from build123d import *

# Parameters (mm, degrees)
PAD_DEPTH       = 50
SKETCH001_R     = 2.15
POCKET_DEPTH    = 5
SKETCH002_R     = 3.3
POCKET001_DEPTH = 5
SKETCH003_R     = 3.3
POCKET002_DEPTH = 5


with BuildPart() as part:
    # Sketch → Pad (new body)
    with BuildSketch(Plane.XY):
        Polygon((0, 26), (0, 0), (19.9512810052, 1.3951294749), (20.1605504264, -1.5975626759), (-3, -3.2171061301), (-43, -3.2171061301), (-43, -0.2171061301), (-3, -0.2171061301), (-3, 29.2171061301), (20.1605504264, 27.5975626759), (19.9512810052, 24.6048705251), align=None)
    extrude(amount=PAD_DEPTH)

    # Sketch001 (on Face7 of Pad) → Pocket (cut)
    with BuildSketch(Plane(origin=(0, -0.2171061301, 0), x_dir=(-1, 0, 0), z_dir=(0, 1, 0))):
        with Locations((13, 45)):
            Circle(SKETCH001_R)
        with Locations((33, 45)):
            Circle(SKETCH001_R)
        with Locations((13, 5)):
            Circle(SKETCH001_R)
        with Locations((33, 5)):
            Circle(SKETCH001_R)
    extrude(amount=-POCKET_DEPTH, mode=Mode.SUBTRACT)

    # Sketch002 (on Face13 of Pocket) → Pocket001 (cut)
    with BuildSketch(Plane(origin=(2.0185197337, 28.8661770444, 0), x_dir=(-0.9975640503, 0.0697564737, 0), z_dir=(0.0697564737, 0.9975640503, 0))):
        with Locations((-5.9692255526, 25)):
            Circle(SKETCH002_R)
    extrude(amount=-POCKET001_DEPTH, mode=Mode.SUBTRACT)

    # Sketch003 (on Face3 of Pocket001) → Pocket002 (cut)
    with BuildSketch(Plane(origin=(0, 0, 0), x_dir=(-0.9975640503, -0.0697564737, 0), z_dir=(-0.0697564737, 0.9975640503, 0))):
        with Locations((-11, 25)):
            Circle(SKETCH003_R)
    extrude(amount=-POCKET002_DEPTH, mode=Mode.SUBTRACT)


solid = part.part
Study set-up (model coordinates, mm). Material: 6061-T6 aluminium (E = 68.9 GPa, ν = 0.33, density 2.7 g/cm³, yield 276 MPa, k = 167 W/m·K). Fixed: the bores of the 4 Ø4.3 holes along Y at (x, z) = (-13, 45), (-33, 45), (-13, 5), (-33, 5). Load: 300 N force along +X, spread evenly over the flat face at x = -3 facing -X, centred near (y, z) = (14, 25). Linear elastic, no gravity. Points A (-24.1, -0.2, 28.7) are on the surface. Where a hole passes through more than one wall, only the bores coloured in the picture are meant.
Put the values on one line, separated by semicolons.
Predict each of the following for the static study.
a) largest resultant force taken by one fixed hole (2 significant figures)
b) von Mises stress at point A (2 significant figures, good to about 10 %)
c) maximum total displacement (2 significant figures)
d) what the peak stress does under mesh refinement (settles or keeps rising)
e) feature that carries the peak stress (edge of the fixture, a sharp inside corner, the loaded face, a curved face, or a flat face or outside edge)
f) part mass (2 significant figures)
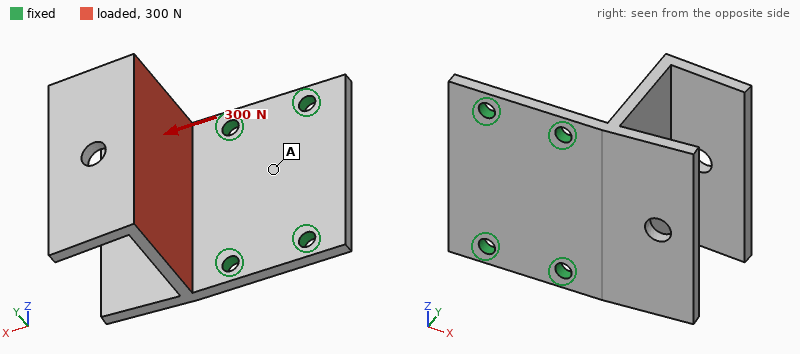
120 N; 9.0 MPa; 0.44 mm; keeps rising; edge of the fixture; 45 g
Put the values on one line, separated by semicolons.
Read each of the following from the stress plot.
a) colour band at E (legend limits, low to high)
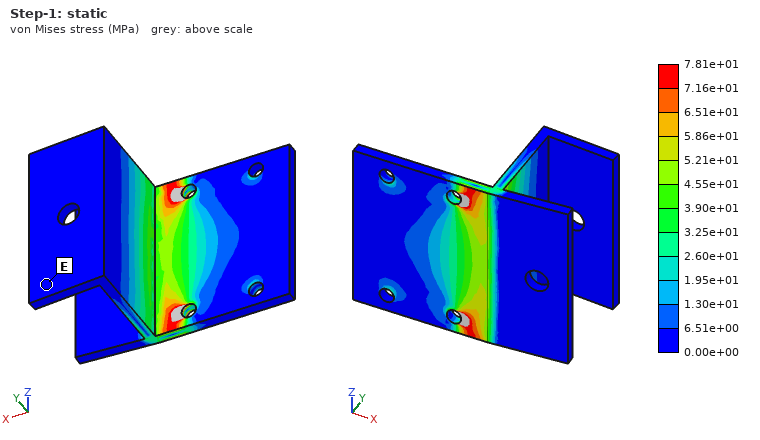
0.00e+00 to 6.51e+00 MPa
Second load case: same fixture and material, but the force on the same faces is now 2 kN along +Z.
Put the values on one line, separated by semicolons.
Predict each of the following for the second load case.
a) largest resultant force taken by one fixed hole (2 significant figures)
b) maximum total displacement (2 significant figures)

1.3 kN; 0.24 mm
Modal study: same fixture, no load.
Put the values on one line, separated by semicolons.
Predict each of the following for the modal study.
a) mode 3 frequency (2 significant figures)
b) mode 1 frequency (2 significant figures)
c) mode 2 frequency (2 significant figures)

3000 Hz; 860 Hz; 2200 Hz
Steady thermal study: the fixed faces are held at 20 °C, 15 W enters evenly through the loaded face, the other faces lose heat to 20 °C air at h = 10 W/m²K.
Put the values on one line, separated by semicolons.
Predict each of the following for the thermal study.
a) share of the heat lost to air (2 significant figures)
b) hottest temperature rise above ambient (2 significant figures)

5.9 %; 17 K
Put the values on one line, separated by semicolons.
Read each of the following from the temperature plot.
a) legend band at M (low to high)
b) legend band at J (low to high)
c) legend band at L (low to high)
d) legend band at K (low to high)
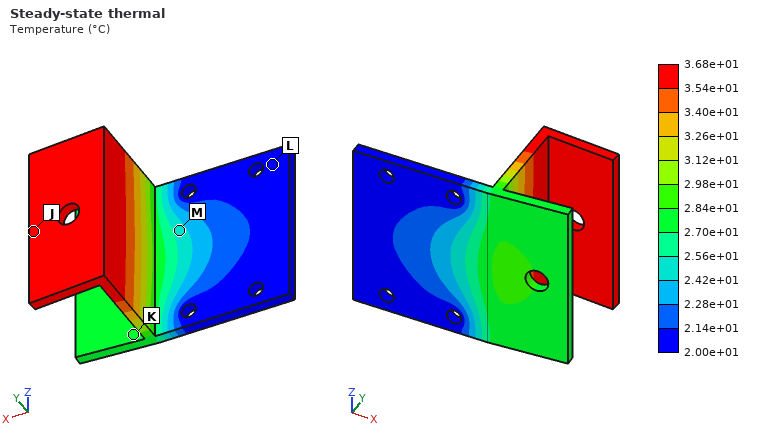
2.42e+01 to 2.56e+01 °C; 3.54e+01 to 3.68e+01 °C; 2.00e+01 to 2.14e+01 °C; 2.70e+01 to 2.84e+01 °C
